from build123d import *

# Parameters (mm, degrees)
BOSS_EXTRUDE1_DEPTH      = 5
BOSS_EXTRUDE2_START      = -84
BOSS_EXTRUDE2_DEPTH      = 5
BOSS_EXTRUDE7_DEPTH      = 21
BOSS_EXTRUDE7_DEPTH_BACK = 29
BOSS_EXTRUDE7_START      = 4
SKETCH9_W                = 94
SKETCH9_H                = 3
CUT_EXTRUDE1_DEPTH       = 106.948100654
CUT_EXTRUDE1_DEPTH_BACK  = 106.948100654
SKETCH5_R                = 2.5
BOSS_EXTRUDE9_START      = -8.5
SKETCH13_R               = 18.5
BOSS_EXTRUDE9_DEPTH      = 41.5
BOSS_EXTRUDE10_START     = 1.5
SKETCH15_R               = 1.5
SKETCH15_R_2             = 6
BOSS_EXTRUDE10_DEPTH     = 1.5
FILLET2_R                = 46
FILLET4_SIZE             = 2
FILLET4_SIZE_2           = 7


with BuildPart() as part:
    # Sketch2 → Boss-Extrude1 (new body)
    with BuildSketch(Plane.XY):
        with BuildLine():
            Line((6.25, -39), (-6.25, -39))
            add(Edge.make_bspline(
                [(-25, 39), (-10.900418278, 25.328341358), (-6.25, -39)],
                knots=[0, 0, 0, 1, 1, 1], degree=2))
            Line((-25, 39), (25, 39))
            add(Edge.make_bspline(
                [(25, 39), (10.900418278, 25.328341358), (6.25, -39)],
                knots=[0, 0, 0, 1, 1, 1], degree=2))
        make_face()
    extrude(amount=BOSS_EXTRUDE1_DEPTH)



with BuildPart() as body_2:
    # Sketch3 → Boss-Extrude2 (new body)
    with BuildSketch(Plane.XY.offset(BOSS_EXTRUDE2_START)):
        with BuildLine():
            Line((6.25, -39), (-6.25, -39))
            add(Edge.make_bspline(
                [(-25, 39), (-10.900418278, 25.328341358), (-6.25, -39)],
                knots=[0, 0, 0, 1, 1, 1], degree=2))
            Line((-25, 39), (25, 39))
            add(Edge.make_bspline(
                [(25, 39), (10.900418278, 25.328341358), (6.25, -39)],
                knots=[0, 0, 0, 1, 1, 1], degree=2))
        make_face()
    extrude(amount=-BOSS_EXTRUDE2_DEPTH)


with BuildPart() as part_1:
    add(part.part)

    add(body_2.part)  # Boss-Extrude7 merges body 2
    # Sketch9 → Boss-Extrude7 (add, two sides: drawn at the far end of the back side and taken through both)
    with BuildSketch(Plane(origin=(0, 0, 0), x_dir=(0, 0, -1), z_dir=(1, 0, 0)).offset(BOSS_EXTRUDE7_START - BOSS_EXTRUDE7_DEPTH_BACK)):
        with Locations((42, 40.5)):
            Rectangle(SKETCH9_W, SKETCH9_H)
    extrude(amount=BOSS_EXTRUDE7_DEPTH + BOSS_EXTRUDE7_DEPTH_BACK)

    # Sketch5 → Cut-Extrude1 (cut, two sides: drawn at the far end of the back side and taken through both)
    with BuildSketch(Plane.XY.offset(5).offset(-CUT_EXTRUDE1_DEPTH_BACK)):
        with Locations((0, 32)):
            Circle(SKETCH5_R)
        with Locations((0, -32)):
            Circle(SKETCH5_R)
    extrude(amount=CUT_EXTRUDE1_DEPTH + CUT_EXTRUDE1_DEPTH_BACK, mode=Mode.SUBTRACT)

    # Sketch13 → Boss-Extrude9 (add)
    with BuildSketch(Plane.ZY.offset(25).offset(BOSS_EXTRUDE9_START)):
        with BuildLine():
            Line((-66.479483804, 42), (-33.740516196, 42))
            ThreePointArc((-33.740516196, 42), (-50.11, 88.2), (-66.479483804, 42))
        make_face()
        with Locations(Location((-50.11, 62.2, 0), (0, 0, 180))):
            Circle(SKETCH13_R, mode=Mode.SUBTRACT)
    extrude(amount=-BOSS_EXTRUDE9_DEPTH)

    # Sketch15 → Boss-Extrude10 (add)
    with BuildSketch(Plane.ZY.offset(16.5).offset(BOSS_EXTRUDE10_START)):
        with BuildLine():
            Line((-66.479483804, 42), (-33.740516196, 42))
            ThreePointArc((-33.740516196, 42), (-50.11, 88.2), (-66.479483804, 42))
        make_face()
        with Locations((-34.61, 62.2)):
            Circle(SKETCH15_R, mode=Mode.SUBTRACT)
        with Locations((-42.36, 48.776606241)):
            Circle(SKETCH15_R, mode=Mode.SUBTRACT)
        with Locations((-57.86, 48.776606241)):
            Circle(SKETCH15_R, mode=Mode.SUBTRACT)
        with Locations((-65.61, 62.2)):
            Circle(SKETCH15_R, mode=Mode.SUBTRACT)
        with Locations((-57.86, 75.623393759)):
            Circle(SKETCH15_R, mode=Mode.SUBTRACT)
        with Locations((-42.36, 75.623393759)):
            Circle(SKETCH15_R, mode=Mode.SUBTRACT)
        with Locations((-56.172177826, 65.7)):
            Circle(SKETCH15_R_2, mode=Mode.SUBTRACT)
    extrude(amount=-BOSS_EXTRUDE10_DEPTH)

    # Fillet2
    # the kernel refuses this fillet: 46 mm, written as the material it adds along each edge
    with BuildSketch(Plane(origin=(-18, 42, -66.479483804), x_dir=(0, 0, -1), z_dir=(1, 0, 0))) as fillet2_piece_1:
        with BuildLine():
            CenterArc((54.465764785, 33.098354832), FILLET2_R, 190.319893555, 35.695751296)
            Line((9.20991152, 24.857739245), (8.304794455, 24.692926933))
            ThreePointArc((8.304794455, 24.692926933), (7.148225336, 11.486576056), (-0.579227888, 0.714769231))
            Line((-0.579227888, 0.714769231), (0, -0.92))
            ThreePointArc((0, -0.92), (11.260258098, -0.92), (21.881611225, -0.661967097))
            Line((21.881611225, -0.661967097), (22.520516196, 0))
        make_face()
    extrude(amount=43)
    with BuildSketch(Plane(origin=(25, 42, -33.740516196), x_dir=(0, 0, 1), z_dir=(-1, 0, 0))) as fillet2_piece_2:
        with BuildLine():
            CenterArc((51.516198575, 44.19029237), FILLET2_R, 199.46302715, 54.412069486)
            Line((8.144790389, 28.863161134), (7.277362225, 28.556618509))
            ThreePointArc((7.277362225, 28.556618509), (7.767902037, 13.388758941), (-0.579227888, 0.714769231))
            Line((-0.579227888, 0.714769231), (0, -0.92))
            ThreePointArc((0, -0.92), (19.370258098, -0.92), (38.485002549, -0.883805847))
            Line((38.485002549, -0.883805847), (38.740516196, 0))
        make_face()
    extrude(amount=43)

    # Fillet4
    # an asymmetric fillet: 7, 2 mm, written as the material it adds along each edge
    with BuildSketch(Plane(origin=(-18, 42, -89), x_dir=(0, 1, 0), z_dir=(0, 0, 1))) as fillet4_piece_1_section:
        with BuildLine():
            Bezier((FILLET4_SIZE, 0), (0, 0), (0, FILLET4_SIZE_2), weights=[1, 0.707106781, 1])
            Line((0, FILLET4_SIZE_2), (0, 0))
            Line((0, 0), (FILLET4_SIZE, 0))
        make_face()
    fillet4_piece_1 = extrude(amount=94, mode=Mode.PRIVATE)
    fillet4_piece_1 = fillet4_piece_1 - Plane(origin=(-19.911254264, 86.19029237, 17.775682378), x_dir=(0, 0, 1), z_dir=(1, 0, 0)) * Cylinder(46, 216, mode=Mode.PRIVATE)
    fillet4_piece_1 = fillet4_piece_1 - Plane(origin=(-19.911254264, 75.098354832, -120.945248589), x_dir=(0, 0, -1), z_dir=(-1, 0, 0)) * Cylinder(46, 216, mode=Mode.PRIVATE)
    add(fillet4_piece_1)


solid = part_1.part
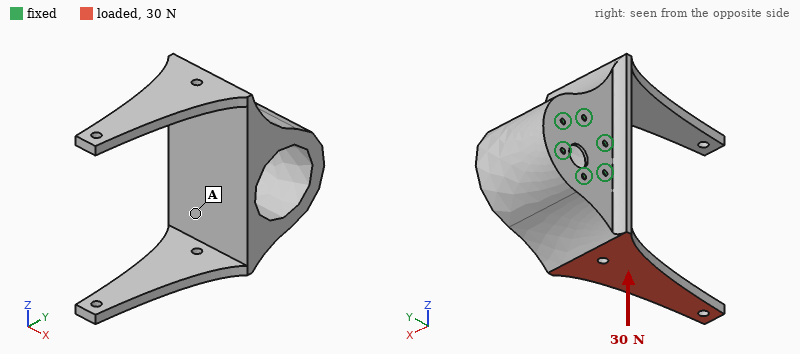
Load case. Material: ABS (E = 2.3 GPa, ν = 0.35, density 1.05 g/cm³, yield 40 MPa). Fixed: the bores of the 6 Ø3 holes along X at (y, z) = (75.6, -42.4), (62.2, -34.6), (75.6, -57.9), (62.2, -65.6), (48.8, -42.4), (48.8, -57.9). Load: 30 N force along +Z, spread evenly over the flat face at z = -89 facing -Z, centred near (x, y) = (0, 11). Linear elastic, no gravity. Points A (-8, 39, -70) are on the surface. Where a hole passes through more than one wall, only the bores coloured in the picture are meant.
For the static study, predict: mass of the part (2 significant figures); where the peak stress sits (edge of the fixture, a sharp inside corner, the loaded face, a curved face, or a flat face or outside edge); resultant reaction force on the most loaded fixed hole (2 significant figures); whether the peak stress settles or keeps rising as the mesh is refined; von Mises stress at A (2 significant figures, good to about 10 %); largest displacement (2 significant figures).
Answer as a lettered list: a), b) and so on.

a) 99 g
b) a sharp inside corner
c) 27 N
d) keeps rising
e) 0.60 MPa
f) 1.9 mm
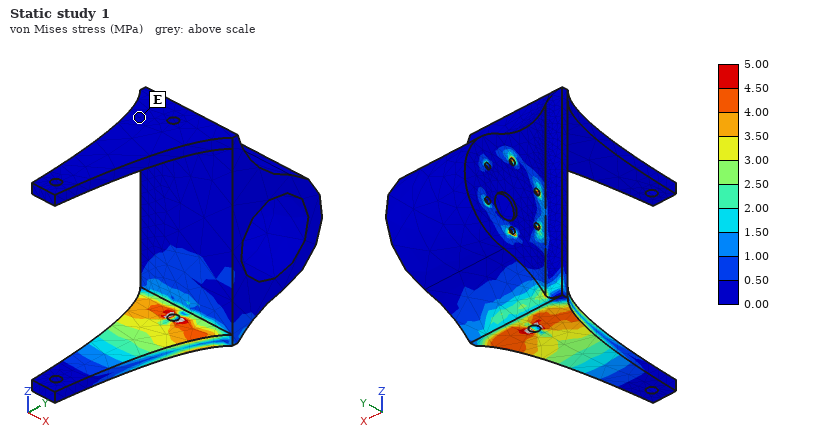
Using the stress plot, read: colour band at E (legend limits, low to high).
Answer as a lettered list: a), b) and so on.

a) 0.00 to 0.50 MPa
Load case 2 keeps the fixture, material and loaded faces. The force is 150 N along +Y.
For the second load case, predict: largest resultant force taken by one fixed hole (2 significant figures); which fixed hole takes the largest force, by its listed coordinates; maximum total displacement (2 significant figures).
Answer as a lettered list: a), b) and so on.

a) 120 N
b) (62.2, -65.6)
c) 1.2 mm
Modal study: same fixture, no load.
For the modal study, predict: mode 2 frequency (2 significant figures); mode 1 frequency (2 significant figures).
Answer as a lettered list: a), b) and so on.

a) 260 Hz
b) 240 Hz
